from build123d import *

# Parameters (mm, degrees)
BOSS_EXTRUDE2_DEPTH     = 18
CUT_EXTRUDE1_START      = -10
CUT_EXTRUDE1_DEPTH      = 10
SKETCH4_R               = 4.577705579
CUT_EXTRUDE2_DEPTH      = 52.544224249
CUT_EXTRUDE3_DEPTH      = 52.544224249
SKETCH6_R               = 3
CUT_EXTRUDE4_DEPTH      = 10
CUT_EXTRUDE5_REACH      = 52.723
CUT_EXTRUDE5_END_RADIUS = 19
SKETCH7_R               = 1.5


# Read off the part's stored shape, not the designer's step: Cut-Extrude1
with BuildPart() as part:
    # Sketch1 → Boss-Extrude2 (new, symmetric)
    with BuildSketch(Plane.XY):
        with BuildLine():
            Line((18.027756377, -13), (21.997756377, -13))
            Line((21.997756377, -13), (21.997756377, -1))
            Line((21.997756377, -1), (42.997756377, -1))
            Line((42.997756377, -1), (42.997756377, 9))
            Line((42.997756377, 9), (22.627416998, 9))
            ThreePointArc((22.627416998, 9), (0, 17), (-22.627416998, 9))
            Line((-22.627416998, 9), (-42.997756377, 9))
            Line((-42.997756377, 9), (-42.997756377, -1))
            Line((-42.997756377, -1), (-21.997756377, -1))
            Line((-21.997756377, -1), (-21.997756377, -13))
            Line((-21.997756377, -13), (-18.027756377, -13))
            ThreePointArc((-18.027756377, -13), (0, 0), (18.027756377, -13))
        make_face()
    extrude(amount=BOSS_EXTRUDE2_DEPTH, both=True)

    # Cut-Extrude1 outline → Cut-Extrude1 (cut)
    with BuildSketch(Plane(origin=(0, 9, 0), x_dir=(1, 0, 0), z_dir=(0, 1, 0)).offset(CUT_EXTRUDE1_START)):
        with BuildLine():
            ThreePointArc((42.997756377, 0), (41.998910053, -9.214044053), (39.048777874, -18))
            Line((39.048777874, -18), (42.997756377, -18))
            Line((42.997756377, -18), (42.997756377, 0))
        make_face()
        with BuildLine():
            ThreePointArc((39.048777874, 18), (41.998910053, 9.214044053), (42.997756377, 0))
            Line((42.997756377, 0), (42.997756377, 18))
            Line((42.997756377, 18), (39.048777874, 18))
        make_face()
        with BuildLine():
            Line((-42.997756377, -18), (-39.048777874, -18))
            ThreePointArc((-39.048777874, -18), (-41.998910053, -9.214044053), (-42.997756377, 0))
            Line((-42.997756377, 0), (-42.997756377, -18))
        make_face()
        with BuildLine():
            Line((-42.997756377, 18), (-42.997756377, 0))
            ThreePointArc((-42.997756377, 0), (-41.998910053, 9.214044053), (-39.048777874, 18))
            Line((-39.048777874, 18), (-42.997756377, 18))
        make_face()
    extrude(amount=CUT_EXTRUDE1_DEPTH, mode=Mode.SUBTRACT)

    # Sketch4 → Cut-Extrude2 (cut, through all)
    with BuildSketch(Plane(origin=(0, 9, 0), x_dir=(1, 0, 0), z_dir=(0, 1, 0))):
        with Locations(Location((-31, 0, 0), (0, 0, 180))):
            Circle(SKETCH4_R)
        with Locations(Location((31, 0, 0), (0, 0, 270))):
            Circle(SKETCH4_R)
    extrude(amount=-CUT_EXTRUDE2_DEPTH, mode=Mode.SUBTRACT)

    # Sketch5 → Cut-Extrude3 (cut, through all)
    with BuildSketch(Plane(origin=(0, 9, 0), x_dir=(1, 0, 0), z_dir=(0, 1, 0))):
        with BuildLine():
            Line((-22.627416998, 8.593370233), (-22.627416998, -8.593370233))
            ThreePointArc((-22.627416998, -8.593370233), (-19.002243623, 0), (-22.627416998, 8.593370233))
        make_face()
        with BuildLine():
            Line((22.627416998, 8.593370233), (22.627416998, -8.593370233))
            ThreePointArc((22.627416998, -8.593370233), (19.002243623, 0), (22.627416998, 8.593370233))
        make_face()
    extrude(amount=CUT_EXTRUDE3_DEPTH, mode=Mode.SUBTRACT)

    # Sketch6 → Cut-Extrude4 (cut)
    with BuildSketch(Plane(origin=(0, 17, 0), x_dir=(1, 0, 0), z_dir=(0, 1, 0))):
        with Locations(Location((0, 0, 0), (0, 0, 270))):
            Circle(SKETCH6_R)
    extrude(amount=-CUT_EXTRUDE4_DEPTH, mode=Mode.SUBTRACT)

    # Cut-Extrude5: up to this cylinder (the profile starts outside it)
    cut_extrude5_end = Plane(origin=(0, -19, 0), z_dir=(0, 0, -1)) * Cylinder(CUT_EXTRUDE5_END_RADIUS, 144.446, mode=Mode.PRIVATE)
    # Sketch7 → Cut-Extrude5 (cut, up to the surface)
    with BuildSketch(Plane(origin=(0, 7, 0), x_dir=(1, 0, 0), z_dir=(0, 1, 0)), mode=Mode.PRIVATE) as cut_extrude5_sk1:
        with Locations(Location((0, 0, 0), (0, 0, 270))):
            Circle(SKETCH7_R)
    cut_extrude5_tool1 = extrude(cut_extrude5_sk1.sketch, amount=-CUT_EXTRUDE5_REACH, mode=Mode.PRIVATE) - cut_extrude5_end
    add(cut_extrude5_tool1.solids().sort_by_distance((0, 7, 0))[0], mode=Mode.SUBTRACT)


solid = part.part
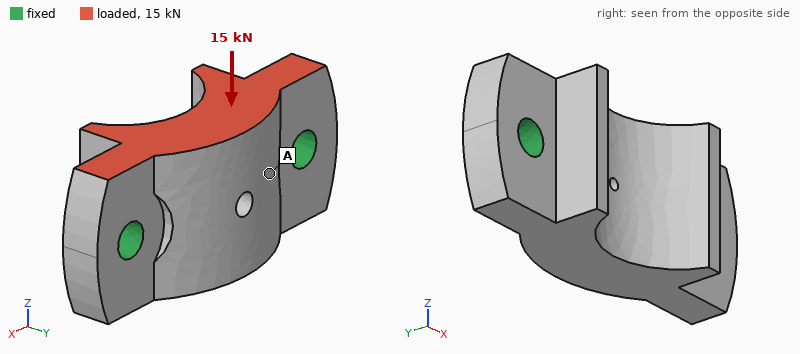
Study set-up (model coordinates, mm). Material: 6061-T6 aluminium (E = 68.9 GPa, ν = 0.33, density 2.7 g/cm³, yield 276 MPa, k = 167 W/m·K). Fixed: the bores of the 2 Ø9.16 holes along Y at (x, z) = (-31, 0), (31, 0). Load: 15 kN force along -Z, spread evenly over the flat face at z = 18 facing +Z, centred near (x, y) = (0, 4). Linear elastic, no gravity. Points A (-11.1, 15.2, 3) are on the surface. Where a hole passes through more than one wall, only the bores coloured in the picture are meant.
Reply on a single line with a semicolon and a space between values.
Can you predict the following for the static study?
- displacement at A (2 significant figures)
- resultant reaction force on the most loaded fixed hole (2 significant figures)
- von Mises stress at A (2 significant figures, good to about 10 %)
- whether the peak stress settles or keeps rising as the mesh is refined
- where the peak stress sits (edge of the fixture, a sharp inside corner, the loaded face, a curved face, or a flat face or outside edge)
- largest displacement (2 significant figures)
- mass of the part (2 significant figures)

17 µm; 7.5 kN; 15 MPa; keeps rising; edge of the fixture; 23 µm; 120 g
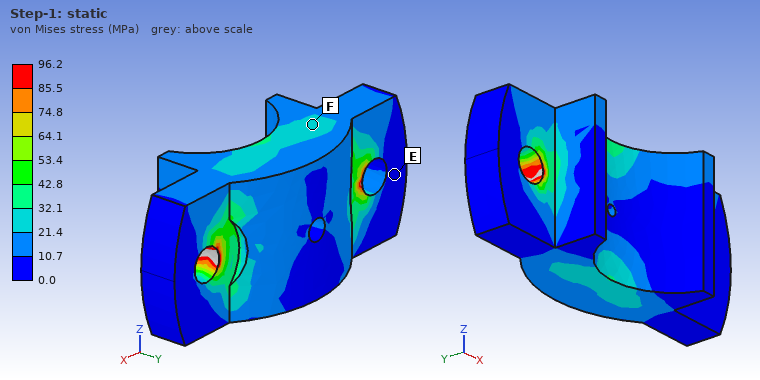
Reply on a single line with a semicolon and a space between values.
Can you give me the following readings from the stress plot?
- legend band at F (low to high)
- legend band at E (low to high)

21.4 to 32.1 MPa; 0.0 to 10.7 MPa
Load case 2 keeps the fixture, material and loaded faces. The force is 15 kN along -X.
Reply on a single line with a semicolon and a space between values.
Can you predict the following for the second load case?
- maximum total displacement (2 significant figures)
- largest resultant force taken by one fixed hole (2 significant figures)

26 µm; 8.4 kN
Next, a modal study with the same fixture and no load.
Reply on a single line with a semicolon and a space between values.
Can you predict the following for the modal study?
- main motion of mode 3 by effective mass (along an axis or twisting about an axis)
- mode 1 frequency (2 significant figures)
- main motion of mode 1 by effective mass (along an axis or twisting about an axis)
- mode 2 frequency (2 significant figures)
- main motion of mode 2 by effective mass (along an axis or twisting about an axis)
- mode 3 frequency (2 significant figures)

along Z; 10 kHz; twisting about X; 12 kHz; along Y; 15 kHz
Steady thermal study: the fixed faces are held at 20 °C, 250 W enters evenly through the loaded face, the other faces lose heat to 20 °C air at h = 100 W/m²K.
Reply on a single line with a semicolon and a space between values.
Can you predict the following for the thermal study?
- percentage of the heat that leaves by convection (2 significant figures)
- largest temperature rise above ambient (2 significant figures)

6.5 %; 42 K
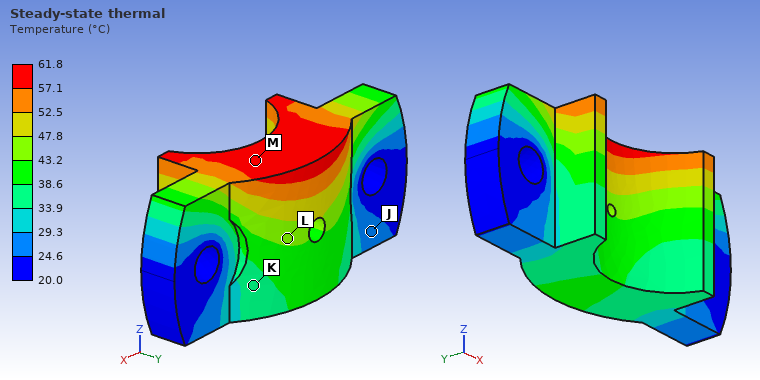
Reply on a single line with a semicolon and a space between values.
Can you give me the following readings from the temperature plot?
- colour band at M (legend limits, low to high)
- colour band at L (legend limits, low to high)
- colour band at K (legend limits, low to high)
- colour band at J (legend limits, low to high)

57.1 to 61.8 °C; 43.2 to 47.8 °C; 33.9 to 38.6 °C; 24.6 to 29.3 °C
